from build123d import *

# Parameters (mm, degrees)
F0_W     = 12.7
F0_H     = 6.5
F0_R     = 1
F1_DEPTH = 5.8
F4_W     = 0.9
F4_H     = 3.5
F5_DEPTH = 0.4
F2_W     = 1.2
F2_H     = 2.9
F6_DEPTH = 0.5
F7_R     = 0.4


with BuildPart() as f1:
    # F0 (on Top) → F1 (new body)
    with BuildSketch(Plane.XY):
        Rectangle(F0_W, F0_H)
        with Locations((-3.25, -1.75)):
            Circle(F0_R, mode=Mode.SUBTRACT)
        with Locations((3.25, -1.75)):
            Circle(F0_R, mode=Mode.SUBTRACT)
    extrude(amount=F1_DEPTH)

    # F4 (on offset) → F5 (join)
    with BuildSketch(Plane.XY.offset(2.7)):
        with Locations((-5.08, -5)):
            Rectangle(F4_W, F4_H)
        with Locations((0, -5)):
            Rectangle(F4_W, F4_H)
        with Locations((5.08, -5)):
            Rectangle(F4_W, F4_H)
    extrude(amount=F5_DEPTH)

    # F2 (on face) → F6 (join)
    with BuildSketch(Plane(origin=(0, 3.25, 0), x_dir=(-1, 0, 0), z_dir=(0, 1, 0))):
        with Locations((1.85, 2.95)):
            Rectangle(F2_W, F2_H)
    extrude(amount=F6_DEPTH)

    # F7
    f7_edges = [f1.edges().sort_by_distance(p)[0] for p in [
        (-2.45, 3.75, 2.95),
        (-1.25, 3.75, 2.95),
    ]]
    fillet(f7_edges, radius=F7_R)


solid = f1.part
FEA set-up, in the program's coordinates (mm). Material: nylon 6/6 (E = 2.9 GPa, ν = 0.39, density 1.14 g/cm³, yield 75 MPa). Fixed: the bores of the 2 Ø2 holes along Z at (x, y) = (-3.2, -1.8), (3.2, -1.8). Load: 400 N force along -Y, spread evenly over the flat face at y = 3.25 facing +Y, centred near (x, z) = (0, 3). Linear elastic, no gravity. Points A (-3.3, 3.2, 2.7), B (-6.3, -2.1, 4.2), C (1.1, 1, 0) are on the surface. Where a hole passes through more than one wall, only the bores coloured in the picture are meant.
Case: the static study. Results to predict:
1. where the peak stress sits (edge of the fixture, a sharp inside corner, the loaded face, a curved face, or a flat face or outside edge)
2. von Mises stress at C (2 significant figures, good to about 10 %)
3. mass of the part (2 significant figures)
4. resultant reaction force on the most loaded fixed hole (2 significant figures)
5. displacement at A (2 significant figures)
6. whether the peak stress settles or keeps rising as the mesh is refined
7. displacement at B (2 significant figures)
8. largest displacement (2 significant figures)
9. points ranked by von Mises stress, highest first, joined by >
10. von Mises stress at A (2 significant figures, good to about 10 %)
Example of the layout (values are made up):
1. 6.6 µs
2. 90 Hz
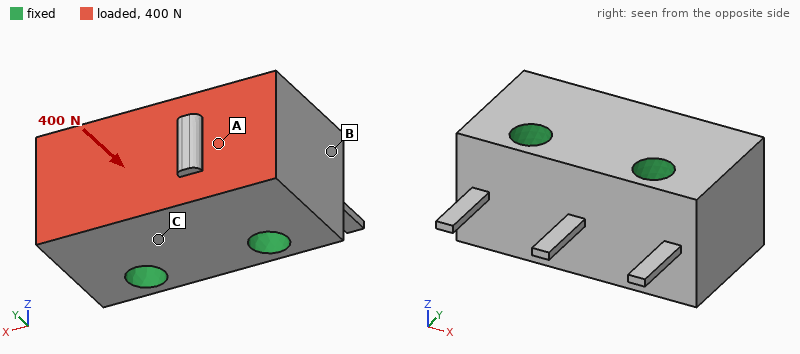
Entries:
1. edge of the fixture
2. 4.3 MPa
3. 0.51 g
4. 210 N
5. 10 µm
6. keeps rising
7. 6.8 µm
8. 15 µm
9. A > C > B
10. 7.0 MPa
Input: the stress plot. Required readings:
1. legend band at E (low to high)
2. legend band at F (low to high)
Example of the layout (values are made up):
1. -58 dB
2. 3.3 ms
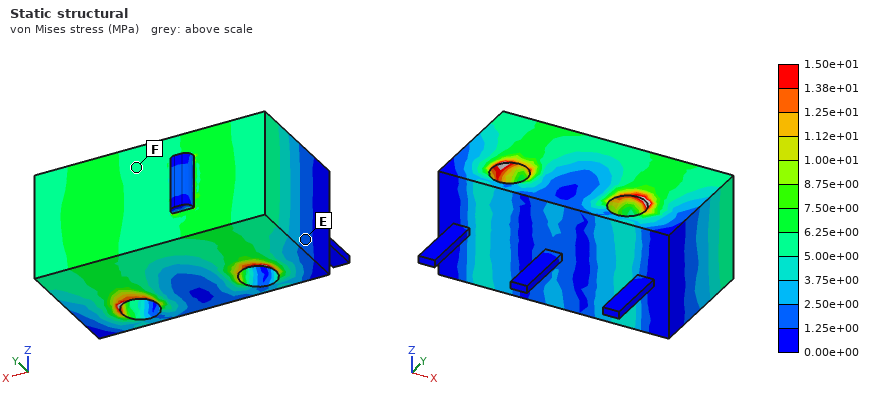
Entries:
1. 1.25e+00 to 2.50e+00 MPa
2. 5.00e+00 to 6.25e+00 MPa
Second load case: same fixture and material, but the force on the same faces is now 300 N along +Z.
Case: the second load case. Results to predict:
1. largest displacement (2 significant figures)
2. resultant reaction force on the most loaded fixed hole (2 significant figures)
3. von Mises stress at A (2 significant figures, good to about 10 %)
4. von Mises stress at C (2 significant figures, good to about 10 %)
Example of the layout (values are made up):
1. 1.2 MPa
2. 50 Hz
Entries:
1. 51 µm
2. 150 N
3. 7.6 MPa
4. 7.9 MPa
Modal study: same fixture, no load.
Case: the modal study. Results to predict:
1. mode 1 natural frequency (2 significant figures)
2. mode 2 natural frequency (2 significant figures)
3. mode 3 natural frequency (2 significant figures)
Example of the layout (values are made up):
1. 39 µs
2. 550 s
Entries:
1. 8100 Hz
2. 8100 Hz
3. 8100 Hz
